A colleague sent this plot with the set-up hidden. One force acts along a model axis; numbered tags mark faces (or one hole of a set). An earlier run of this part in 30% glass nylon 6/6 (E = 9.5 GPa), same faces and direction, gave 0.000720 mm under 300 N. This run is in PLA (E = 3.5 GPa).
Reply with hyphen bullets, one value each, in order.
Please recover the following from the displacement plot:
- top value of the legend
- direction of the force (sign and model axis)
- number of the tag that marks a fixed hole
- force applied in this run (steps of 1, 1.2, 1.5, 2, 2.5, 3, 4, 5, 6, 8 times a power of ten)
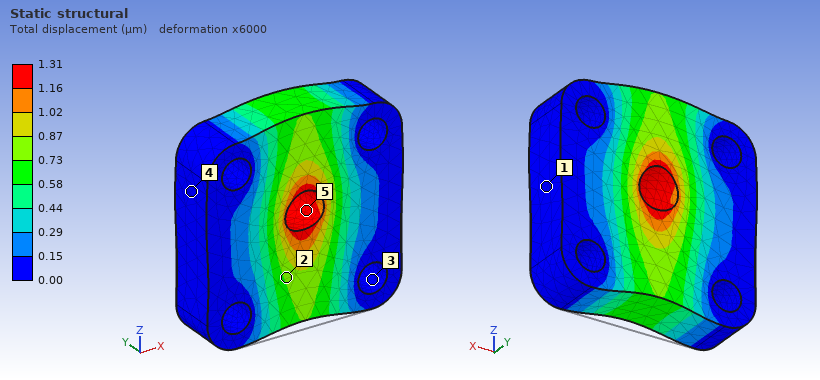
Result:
- 1.31 µm
- +Z
- 3
- 200 N
